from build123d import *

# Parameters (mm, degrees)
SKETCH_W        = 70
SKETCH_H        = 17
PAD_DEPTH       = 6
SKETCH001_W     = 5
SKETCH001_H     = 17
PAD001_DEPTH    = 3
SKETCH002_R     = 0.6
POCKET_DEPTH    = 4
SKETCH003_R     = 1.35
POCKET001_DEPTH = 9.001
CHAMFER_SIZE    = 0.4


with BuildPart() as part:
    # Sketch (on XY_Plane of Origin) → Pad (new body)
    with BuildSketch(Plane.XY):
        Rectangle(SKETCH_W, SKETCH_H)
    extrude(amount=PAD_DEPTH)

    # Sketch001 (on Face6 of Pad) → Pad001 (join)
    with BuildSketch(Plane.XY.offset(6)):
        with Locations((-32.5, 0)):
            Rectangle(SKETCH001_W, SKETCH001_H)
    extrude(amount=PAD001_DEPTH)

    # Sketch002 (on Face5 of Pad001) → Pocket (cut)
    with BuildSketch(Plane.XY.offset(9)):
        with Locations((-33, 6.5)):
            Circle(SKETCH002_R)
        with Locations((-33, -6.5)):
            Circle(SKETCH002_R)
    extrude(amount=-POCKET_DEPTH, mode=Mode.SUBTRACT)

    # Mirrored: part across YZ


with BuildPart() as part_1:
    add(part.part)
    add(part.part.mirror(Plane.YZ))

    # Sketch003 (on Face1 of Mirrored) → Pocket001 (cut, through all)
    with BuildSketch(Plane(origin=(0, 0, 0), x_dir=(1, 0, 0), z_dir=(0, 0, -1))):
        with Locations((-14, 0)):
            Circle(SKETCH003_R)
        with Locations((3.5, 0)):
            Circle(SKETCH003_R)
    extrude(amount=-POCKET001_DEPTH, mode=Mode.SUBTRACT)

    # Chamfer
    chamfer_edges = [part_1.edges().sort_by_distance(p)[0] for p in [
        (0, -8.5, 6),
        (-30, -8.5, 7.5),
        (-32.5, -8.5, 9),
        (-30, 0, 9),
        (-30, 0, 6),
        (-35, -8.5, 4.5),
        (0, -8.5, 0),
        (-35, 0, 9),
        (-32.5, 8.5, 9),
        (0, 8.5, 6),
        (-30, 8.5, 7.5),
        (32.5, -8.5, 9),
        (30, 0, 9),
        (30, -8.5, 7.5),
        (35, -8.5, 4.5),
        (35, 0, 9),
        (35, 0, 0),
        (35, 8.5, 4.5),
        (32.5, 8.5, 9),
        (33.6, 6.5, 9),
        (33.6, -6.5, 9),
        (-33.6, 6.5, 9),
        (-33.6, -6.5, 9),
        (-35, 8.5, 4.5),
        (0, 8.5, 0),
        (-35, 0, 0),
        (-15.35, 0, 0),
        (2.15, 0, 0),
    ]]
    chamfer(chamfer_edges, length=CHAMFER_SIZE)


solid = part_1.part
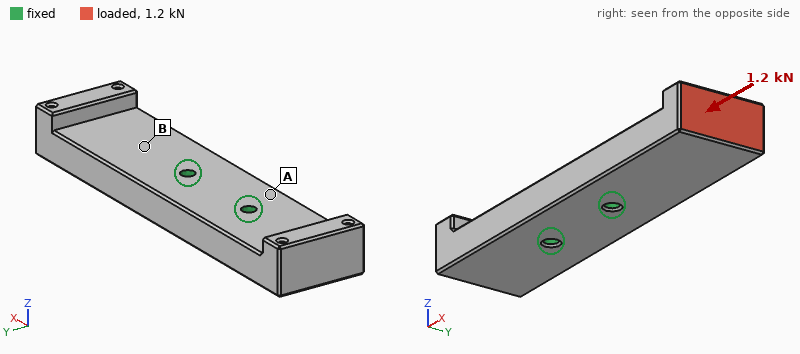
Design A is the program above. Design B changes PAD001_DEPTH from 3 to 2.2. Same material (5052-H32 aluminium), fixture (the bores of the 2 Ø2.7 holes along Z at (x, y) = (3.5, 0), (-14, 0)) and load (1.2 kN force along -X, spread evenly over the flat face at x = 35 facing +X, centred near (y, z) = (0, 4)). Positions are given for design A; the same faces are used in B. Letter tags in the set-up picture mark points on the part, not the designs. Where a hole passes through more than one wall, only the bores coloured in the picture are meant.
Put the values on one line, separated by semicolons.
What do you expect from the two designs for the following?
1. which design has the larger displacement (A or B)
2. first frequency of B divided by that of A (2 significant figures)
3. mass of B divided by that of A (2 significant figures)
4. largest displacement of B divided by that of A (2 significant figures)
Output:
A; 1.0; 0.98; 0.73
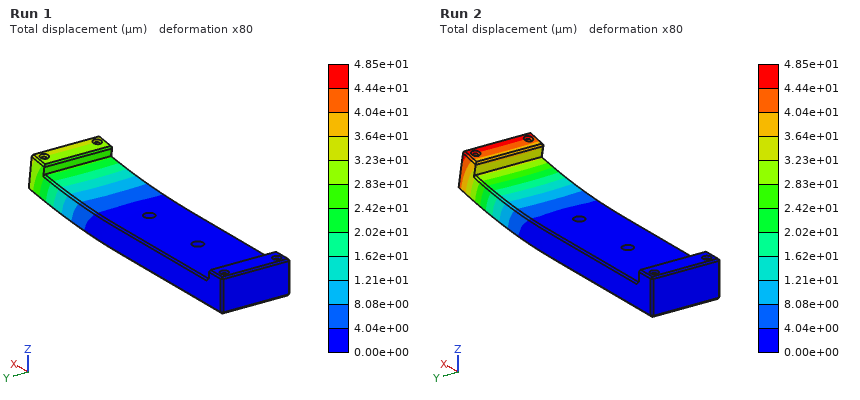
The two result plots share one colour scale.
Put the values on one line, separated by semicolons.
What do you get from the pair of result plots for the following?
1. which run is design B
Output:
Run 1
